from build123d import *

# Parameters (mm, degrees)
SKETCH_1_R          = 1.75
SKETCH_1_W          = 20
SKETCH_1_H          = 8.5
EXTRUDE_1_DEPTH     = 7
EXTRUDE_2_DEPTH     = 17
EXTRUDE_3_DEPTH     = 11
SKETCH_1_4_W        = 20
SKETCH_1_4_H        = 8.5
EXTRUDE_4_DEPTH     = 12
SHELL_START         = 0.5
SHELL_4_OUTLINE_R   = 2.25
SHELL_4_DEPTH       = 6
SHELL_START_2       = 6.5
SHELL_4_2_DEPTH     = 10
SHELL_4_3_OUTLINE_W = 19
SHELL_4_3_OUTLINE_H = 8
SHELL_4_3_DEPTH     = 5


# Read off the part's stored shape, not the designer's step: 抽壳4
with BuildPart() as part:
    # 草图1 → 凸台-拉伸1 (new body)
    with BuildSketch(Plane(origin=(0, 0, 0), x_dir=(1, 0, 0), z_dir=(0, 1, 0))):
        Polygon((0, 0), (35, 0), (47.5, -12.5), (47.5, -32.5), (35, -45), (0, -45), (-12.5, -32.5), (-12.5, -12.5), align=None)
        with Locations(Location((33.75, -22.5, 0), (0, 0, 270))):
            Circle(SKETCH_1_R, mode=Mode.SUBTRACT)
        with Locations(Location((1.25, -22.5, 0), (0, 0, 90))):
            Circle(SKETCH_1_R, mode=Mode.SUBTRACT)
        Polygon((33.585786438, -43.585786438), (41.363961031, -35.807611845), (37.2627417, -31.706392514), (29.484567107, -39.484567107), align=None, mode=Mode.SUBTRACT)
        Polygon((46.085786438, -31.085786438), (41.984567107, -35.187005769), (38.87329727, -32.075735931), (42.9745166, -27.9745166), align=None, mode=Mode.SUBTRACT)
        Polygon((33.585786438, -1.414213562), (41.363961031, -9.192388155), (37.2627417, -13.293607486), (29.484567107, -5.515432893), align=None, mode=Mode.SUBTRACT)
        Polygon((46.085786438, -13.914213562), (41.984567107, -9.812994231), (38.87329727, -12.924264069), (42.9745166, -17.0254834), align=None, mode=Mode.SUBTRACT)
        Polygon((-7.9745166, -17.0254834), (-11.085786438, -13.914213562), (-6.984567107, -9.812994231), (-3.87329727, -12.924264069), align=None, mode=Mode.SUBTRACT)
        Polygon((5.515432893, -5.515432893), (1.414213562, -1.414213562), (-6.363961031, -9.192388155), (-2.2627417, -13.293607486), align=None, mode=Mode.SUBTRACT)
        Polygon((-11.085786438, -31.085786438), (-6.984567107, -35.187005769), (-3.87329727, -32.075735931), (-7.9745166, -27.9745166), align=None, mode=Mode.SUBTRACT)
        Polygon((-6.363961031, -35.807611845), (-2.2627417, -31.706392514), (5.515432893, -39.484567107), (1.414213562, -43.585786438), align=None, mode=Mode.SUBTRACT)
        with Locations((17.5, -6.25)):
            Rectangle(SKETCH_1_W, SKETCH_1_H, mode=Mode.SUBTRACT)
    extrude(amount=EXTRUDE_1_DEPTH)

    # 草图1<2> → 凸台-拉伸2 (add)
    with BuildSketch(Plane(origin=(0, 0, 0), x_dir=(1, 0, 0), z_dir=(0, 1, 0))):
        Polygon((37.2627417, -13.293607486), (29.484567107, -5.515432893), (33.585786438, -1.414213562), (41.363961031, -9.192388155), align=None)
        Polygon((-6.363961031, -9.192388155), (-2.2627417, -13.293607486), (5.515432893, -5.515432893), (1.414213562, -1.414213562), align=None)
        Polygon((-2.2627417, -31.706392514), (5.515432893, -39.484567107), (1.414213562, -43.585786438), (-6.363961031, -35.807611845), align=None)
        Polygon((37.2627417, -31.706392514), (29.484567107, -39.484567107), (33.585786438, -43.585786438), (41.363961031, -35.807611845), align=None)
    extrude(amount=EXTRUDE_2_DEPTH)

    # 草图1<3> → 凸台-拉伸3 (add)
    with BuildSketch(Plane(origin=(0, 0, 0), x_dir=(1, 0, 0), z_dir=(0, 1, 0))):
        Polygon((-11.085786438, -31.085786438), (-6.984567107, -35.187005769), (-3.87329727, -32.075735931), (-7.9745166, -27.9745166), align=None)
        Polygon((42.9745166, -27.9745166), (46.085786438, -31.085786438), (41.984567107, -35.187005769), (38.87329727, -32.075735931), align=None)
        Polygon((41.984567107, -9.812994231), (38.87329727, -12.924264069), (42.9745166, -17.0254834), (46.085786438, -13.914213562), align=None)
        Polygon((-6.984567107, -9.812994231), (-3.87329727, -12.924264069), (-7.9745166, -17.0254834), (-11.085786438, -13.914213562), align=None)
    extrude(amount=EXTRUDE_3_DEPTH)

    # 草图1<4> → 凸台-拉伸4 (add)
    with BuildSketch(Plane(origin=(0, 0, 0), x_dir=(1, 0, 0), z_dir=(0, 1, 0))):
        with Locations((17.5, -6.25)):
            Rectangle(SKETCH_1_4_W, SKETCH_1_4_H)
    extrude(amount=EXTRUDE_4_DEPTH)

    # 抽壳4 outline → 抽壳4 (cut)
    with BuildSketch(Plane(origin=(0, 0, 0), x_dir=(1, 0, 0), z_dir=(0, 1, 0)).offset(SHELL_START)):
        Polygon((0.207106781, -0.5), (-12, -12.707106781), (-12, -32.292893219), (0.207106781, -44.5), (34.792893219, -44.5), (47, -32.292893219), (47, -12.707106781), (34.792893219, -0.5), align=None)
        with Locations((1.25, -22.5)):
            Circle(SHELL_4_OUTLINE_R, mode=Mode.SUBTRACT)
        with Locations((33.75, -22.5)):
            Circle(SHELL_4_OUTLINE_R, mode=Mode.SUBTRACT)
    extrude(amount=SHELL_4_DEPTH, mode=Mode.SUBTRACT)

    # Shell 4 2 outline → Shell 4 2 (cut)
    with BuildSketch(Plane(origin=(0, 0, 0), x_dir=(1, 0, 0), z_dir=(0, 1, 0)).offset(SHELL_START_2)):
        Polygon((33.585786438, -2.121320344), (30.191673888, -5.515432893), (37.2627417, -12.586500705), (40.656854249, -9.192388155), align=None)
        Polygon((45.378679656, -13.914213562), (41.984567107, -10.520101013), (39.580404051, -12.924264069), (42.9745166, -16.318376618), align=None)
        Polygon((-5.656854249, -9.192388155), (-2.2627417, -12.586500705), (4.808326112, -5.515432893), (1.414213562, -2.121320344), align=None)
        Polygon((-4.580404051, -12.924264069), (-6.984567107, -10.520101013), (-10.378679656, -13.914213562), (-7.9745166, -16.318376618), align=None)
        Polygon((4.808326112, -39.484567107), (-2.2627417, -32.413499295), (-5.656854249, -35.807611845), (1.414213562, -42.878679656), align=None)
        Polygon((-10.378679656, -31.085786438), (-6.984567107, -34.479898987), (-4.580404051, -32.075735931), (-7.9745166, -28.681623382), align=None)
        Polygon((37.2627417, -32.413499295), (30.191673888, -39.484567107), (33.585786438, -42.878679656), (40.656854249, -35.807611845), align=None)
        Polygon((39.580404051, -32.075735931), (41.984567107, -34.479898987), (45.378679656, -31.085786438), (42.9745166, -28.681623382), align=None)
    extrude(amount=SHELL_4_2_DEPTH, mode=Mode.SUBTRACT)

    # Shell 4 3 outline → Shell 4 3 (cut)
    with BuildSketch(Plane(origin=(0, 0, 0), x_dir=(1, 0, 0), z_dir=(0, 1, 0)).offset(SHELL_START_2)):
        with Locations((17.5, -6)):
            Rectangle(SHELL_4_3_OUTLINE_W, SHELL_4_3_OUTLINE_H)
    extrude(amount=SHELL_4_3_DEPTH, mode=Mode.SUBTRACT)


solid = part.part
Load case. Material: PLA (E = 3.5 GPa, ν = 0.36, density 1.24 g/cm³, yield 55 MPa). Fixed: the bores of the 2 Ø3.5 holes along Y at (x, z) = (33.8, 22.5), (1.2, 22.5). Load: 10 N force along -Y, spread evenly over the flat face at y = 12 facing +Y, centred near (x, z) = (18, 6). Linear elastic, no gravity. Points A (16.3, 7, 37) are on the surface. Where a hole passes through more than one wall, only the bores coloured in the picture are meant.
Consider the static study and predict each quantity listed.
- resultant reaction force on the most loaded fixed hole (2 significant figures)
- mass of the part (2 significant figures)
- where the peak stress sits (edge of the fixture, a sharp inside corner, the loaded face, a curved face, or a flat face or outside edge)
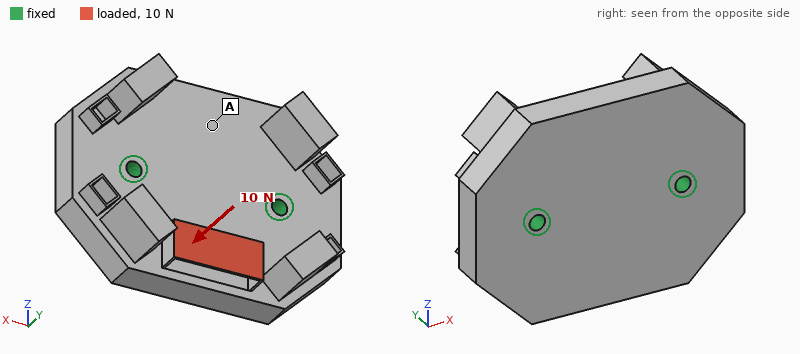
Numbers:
5.1 N
4.7 g
a flat face or outside edge
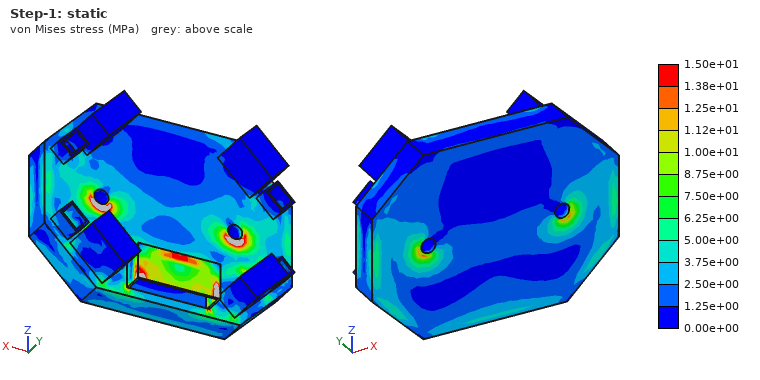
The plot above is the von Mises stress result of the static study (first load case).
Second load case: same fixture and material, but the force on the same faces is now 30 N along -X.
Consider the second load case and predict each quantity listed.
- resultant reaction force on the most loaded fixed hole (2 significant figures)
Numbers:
21 N
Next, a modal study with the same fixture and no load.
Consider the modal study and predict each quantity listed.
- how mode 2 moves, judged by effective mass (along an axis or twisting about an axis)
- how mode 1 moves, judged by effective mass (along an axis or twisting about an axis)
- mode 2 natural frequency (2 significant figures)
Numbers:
twisting about X
along Y
790 Hz
